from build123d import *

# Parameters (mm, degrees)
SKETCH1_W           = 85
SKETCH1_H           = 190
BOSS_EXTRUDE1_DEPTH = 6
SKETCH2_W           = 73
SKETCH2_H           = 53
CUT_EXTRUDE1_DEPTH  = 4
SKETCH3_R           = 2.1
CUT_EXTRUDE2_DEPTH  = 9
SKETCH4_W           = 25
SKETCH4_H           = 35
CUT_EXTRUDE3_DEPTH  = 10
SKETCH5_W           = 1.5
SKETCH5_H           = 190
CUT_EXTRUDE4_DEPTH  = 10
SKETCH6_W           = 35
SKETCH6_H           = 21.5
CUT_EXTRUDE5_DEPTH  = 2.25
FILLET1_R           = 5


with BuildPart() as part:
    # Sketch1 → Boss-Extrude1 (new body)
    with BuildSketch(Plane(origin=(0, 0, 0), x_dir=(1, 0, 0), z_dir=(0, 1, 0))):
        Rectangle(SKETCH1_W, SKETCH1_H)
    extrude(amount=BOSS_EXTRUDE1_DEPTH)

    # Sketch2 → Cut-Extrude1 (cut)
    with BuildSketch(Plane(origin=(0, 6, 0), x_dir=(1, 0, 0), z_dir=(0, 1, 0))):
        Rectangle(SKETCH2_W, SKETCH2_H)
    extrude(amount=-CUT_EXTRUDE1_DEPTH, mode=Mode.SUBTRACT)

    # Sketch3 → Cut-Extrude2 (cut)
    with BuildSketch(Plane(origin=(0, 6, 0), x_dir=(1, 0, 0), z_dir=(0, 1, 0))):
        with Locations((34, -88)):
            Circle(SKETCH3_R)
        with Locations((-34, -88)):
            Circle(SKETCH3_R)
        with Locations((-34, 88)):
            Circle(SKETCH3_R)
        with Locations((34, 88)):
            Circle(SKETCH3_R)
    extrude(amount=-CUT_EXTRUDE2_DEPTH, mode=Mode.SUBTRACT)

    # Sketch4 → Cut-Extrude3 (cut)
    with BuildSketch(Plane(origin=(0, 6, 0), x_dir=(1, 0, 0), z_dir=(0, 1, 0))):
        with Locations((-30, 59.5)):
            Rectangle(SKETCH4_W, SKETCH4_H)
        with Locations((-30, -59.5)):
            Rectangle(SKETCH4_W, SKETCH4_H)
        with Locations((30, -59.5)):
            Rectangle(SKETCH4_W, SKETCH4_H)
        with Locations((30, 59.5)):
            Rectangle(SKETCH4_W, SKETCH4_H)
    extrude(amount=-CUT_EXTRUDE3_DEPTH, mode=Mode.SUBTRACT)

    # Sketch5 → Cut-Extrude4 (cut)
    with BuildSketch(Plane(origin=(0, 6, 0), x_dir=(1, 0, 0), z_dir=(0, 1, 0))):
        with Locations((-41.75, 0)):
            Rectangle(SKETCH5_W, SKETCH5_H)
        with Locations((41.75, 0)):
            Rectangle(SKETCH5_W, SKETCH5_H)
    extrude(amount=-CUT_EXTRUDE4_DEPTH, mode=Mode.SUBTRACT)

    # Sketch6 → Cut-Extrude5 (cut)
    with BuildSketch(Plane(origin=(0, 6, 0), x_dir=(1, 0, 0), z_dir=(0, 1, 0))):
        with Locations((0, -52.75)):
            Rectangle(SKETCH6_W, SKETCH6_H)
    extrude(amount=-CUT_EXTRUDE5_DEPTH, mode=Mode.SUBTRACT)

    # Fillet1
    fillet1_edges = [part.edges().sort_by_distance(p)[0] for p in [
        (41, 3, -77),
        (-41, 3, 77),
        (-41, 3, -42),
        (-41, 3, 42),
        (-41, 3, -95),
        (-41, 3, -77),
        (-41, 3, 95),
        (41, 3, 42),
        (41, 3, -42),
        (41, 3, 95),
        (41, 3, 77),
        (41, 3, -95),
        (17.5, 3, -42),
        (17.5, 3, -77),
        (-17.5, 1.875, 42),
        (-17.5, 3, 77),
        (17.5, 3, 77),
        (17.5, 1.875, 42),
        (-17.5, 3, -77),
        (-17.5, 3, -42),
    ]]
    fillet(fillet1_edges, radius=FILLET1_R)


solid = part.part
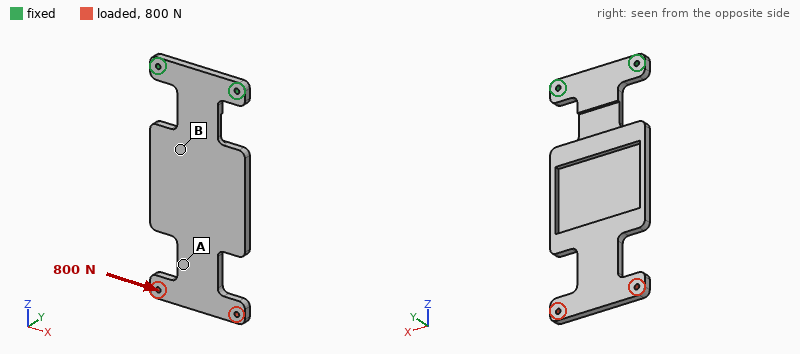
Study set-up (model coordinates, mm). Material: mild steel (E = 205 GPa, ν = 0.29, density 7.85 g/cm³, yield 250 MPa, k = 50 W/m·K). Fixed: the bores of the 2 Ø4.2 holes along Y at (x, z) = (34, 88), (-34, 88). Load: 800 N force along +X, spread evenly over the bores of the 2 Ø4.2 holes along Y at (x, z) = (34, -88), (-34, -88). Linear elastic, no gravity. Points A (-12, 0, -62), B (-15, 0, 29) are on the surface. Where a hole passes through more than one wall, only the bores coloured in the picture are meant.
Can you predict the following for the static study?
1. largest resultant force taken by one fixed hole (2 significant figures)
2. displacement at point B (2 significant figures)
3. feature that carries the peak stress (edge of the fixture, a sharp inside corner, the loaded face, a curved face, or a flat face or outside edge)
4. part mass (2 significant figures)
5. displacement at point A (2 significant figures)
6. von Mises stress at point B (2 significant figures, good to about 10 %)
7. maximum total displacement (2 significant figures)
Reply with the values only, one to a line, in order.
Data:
2.3 kN
0.079 mm
a curved face
440 g
0.29 mm
47 MPa
0.41 mm
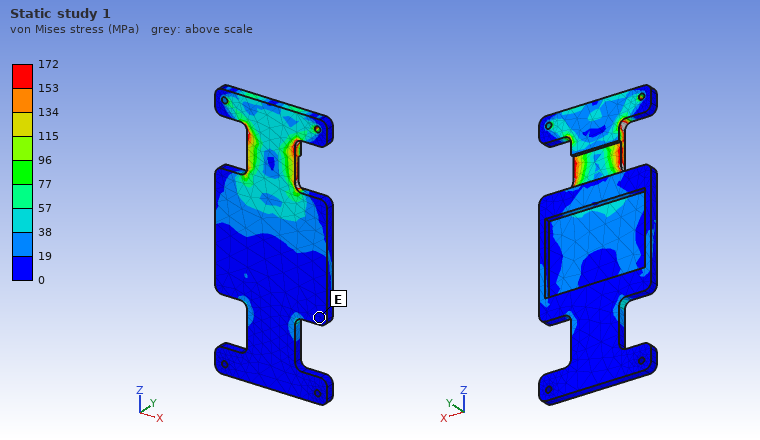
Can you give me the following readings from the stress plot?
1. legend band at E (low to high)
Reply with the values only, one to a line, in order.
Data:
0 to 19 MPa
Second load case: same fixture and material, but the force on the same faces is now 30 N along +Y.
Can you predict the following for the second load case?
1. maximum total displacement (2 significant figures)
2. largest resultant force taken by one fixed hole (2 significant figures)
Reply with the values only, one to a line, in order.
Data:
1.00 mm
15 N
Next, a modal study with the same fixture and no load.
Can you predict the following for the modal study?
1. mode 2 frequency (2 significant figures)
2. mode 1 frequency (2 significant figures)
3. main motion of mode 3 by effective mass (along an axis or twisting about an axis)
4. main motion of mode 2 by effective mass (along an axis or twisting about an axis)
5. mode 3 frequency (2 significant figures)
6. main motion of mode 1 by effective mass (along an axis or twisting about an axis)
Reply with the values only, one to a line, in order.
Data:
430 Hz
78 Hz
along Y
twisting about Z
560 Hz
along Y
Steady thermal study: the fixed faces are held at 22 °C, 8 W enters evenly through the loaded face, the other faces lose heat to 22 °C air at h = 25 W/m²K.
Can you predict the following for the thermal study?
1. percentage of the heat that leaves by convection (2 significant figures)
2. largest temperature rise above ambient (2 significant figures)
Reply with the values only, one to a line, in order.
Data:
96 %
44 K
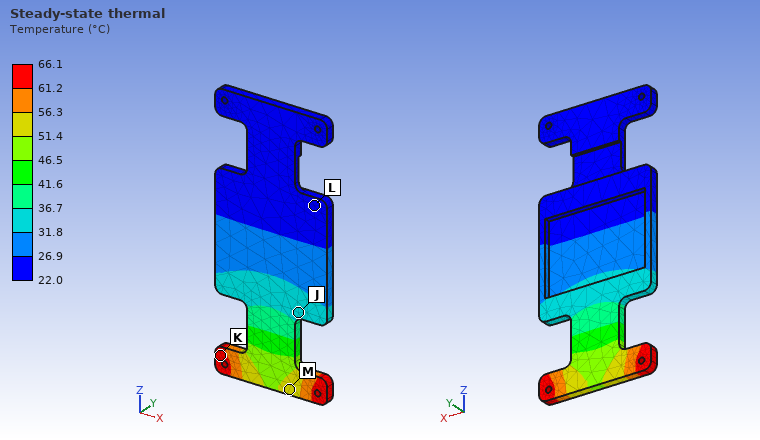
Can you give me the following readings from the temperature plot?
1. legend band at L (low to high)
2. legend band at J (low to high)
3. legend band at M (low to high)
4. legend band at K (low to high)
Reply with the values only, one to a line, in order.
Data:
22.0 to 26.9 °C
31.8 to 36.7 °C
51.4 to 56.3 °C
61.2 to 66.1 °C
